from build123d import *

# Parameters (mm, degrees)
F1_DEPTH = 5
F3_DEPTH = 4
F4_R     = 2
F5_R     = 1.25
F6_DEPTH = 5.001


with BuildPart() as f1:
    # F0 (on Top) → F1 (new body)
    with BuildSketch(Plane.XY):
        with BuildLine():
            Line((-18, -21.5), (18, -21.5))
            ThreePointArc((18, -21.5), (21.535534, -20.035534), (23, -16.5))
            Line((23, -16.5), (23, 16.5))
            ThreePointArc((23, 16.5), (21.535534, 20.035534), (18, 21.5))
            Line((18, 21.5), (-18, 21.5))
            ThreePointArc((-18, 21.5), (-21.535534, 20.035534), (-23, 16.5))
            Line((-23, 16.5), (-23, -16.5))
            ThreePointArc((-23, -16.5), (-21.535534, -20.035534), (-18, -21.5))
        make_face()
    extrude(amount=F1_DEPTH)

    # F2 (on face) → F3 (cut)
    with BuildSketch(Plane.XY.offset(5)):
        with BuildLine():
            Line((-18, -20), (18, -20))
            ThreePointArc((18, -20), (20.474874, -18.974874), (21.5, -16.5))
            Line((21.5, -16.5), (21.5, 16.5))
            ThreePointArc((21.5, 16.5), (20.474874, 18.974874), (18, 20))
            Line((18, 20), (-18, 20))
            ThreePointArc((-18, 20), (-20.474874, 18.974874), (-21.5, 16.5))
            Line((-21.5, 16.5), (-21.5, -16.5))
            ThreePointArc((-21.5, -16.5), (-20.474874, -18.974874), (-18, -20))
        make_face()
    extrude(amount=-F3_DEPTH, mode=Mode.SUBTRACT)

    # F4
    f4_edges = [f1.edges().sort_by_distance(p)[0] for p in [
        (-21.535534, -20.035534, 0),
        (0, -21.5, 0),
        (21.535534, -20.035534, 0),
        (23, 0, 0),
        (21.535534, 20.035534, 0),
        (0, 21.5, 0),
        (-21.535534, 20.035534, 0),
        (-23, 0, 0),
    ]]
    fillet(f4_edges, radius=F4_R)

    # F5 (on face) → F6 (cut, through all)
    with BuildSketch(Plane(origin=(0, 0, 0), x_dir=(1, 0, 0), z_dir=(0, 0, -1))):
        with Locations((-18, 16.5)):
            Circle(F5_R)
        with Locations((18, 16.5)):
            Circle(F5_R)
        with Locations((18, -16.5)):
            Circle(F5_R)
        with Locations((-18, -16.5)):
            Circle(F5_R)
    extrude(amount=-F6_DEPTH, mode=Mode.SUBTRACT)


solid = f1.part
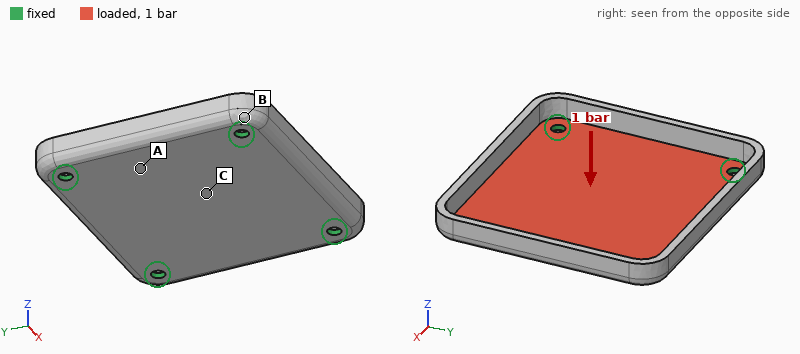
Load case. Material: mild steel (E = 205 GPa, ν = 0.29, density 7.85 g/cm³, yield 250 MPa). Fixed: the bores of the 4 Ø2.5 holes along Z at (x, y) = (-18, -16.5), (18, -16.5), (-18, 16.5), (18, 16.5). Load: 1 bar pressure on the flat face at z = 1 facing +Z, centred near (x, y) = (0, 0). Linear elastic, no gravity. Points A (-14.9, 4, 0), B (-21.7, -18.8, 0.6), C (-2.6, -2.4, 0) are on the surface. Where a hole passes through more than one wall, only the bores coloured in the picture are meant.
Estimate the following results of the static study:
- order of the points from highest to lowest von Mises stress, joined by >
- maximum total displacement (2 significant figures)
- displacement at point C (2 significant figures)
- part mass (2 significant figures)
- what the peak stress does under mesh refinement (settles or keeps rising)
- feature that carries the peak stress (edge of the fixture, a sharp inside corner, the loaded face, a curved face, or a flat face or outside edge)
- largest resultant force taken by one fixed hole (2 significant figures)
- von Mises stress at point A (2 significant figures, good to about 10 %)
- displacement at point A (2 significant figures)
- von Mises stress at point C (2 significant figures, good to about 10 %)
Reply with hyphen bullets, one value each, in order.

- C > A > B
- 34 µm
- 33 µm
- 22 g
- keeps rising
- edge of the fixture
- 47 N
- 16 MPa
- 14 µm
- 31 MPa
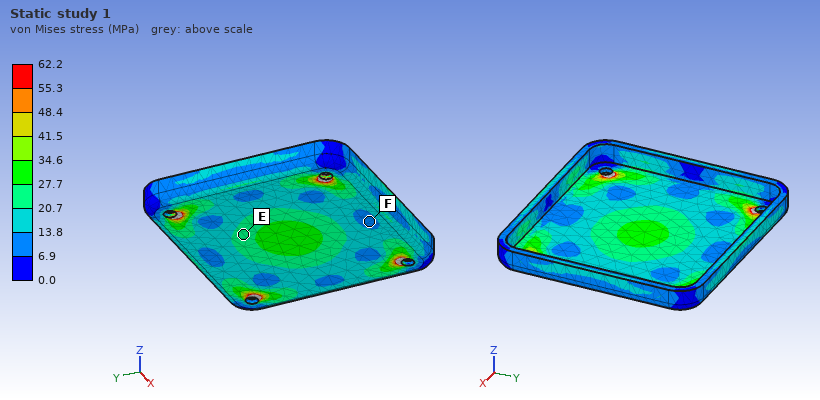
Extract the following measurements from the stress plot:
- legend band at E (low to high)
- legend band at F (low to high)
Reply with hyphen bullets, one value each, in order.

- 20.7 to 27.7 MPa
- 6.9 to 13.8 MPa
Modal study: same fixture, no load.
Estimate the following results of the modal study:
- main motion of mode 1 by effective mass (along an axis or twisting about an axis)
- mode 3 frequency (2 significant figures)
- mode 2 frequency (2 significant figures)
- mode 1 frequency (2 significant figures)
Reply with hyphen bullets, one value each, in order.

- along Z
- 7900 Hz
- 7900 Hz
- 3900 Hz
